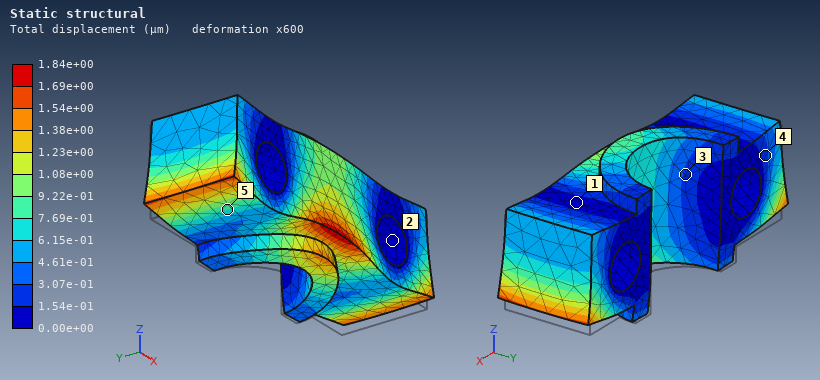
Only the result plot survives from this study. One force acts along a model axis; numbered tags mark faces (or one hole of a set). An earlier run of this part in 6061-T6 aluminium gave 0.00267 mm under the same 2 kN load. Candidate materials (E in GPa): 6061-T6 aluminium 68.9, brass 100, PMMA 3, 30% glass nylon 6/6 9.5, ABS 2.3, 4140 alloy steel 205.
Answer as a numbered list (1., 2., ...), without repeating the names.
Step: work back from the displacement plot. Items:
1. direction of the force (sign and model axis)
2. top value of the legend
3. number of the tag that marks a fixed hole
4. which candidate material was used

1. +Z
2. 1.84e+00 µm
3. 2
4. brass
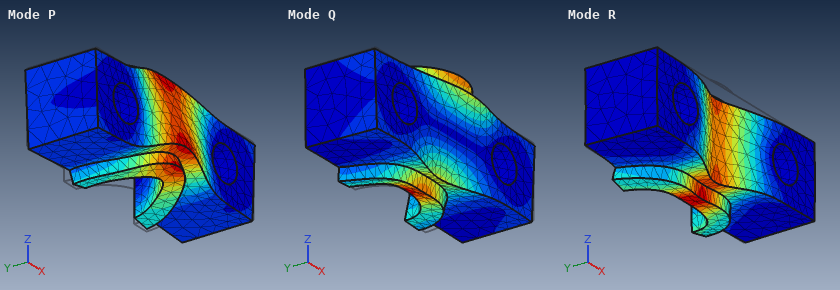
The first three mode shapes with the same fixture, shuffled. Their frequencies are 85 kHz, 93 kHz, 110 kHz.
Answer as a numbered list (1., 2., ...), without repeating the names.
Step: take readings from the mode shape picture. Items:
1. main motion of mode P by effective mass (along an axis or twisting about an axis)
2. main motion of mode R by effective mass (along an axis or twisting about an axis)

1. along Z
2. along Y
